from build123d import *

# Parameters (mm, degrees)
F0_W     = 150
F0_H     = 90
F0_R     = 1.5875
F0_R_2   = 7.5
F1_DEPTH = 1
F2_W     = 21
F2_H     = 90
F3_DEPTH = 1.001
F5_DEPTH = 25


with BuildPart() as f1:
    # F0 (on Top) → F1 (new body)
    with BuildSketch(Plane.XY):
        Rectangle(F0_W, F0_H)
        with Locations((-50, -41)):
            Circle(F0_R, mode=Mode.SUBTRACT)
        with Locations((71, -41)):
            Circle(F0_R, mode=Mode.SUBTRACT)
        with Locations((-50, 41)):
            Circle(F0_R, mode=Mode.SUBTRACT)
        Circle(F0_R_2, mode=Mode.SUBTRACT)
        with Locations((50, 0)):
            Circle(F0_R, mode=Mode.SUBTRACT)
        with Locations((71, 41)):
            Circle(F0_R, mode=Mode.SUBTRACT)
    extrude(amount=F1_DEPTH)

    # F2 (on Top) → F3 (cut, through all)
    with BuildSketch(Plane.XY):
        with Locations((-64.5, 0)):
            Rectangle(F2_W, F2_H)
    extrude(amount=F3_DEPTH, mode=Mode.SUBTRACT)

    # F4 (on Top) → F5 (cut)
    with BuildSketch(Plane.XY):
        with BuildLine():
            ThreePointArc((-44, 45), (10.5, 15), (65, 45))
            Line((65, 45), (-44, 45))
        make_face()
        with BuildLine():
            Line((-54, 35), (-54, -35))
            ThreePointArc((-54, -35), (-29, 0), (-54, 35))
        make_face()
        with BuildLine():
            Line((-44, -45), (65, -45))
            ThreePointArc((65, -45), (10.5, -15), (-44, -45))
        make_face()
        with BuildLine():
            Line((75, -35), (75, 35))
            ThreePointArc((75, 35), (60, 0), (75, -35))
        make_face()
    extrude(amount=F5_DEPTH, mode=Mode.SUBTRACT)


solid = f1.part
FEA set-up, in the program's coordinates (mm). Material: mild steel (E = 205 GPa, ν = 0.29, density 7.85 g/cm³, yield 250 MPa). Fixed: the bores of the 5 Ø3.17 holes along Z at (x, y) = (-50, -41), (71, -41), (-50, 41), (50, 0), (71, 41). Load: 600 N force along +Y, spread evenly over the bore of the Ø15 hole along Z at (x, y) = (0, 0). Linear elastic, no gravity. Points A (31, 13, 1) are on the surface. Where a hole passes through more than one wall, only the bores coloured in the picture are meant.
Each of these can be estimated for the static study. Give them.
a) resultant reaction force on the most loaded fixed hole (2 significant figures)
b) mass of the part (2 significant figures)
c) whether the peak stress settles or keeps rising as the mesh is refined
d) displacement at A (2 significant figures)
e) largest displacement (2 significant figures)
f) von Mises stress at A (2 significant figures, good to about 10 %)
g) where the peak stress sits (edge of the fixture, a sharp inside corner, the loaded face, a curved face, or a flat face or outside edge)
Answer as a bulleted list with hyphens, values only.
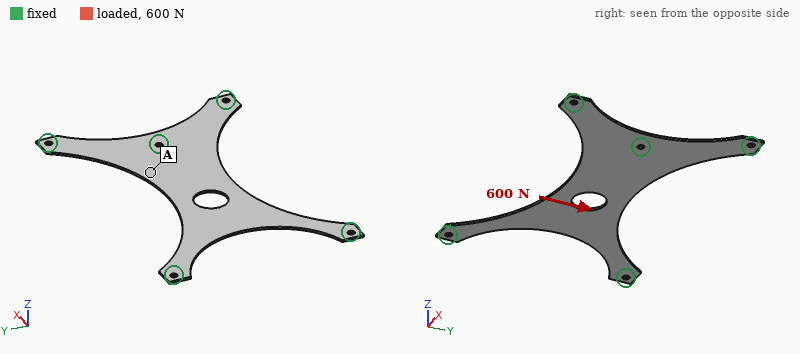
- 260 N
- 37 g
- keeps rising
- 4.5 µm
- 11 µm
- 11 MPa
- edge of the fixture
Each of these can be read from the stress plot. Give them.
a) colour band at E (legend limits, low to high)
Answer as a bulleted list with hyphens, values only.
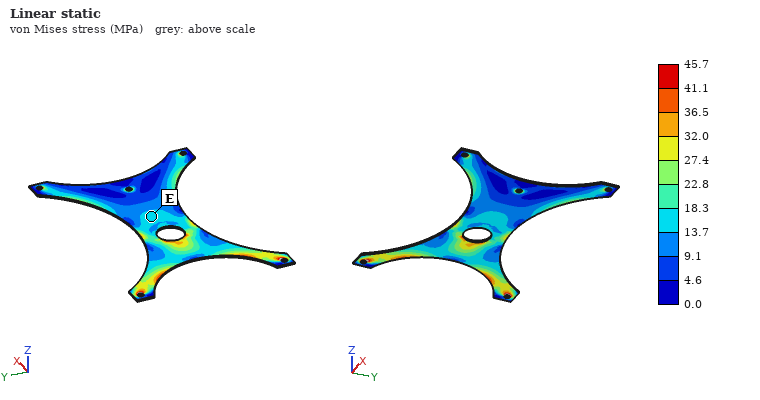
- 13.7 to 18.3 MPa
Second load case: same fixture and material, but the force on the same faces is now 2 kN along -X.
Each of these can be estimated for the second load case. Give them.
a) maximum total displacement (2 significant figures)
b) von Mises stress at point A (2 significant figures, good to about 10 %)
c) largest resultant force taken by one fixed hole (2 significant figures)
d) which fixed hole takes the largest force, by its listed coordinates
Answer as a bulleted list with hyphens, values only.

- 15 µm
- 34 MPa
- 1.1 kN
- (50, 0)
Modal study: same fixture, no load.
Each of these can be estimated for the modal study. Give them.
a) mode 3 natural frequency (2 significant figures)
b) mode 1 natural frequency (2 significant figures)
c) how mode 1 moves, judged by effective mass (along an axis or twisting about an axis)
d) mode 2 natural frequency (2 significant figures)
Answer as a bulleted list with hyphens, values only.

- 1000 Hz
- 420 Hz
- along Z
- 1000 Hz
